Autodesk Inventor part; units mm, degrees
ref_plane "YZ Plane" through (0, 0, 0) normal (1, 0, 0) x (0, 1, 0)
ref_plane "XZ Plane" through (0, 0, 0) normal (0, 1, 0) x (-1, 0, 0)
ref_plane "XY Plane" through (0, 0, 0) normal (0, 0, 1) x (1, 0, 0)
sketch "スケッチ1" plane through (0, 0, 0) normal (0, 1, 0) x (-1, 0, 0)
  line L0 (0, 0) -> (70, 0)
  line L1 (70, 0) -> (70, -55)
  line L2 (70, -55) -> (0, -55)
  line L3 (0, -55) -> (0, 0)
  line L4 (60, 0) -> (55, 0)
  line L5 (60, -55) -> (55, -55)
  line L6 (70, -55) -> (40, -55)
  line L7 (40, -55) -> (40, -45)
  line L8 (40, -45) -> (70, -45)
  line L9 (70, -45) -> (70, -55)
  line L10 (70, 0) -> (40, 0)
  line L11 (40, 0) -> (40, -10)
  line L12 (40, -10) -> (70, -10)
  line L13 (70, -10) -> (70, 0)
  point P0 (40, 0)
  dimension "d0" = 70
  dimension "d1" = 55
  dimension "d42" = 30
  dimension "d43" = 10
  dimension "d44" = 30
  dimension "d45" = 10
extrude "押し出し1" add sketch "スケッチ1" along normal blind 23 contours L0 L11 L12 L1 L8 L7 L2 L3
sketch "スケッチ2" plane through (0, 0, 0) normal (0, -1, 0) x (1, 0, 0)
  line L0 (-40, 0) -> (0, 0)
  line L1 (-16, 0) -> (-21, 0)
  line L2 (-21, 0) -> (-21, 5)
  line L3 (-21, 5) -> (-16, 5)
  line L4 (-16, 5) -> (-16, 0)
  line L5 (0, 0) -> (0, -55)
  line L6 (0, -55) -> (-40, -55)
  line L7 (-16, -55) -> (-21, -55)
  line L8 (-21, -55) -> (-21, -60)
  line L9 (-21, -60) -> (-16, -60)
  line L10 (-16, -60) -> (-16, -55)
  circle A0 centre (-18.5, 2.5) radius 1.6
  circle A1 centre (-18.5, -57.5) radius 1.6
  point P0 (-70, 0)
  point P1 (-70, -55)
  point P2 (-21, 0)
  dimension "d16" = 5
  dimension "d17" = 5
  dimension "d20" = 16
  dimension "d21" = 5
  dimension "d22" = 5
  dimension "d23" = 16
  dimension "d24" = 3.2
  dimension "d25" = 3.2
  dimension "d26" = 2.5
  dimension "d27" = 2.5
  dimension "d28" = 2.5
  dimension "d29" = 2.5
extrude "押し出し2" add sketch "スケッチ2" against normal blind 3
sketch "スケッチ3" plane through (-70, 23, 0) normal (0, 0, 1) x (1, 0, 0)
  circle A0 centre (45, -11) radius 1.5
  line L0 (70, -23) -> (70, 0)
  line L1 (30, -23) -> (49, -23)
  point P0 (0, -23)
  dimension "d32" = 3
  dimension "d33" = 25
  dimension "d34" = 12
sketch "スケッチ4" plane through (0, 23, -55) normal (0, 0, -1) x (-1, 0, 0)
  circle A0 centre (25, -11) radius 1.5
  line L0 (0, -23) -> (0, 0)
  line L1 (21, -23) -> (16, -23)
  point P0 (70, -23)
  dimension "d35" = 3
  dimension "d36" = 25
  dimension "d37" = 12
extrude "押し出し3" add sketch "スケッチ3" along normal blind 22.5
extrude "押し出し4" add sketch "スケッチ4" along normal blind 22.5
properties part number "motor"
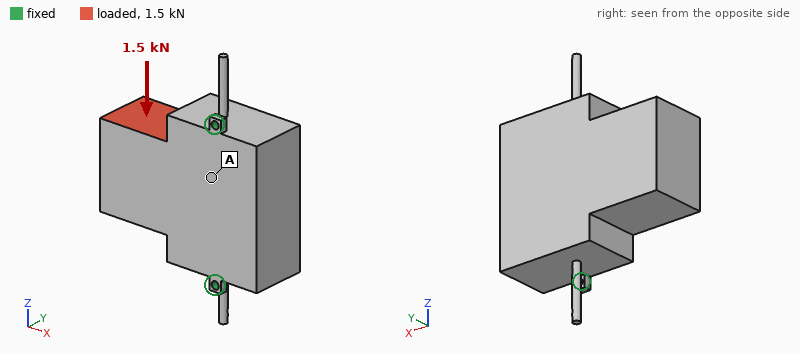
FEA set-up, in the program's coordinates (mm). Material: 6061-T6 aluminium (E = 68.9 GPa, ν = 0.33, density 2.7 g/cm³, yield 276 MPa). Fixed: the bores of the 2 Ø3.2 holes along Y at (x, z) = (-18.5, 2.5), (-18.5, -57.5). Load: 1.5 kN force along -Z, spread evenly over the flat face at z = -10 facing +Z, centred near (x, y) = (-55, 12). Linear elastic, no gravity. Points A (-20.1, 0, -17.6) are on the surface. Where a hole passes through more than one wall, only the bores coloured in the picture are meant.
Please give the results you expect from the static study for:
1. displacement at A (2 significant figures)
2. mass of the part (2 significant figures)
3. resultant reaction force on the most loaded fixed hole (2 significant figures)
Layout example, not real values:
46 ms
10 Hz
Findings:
4.7 µm
200 g
1.3 kN
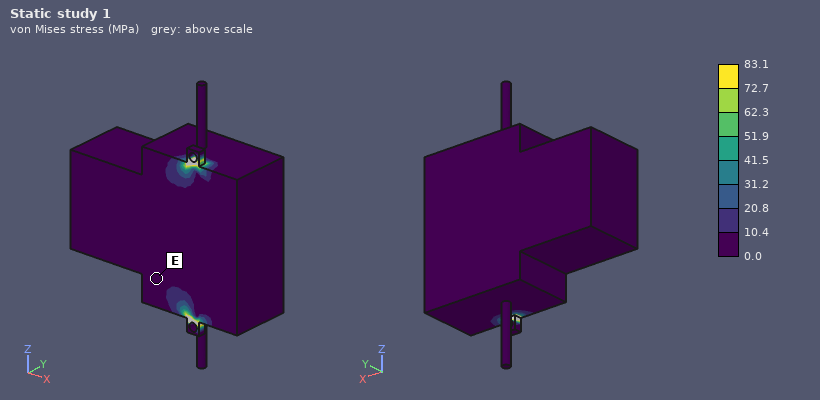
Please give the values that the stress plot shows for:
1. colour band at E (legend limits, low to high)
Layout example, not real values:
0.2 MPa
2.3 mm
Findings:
0.0 to 10.4 MPa
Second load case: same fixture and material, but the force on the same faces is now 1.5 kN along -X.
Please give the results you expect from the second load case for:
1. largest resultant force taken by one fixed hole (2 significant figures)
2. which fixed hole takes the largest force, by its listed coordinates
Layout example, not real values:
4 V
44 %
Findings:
1.2 kN
(-18.5, 2.5)
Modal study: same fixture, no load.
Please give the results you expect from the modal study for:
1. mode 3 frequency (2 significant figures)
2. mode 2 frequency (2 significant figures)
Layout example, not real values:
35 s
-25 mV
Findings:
3900 Hz
3900 Hz
